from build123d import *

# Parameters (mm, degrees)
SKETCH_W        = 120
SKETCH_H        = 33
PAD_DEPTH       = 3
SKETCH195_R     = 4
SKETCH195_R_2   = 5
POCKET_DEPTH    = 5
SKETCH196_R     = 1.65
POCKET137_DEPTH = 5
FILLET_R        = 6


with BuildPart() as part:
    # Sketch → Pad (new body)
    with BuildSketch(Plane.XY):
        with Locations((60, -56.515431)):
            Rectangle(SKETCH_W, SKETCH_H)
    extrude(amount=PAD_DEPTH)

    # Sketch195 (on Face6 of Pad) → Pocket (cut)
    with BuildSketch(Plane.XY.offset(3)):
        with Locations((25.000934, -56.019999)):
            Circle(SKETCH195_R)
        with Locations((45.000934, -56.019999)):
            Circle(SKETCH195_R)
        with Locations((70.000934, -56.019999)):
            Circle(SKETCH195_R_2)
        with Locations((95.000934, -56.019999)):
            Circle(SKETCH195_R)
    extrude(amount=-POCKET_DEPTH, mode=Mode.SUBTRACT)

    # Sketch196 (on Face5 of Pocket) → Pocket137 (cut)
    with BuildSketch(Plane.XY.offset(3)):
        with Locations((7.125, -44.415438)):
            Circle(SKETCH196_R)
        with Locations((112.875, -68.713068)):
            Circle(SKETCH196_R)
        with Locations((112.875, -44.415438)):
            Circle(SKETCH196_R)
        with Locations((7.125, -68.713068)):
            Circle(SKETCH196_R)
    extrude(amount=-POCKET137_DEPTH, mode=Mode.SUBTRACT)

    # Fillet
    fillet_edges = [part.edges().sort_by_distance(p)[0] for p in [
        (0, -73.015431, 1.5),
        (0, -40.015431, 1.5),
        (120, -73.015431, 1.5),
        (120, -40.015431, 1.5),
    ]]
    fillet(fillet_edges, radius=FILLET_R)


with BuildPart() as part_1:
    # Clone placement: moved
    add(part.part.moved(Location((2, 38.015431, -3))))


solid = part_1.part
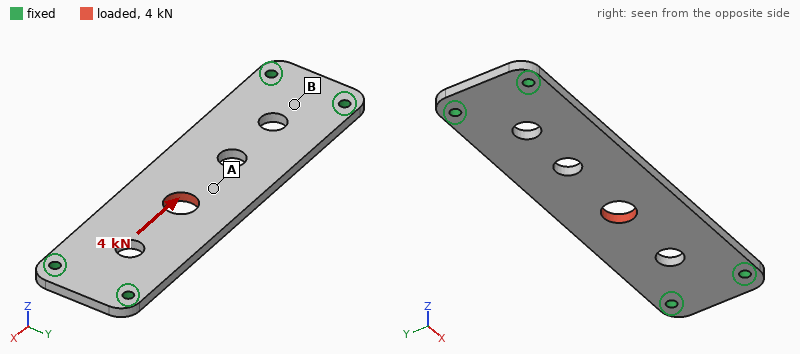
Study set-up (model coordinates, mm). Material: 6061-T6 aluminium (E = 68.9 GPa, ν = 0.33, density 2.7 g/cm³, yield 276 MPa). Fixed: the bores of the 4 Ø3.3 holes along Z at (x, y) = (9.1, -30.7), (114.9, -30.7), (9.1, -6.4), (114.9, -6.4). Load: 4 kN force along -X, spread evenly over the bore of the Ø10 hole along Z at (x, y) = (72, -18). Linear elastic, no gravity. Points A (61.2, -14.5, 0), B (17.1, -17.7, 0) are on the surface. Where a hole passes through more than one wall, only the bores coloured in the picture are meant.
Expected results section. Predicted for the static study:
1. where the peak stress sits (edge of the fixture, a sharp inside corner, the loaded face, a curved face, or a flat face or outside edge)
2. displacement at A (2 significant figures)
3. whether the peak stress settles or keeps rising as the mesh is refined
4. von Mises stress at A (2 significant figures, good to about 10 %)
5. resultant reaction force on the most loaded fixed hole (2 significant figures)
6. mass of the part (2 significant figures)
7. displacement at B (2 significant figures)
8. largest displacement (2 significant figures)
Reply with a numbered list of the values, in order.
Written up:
1. edge of the fixture
2. 18 µm
3. keeps rising
4. 31 MPa
5. 1.2 kN
6. 30 g
7. 3.3 µm
8. 21 µm
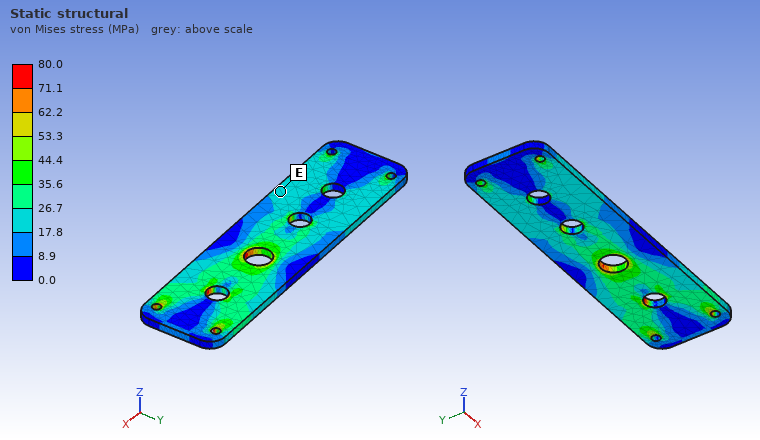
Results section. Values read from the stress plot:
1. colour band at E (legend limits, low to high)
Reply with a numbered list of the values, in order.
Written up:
1. 17.8 to 26.7 MPa
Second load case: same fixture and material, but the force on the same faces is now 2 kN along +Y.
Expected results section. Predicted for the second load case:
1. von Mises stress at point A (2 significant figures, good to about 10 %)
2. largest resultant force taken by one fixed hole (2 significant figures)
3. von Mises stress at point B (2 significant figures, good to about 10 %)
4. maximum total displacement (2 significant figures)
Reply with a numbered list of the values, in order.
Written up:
1. 18 MPa
2. 1.3 kN
3. 24 MPa
4. 49 µm
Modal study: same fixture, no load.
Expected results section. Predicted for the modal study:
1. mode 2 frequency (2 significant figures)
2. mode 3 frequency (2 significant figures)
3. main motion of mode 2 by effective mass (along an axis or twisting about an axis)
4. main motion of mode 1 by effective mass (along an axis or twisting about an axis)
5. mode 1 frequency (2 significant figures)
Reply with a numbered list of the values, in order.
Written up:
1. 3000 Hz
2. 3800 Hz
3. twisting about X
4. along Z
5. 1400 Hz
